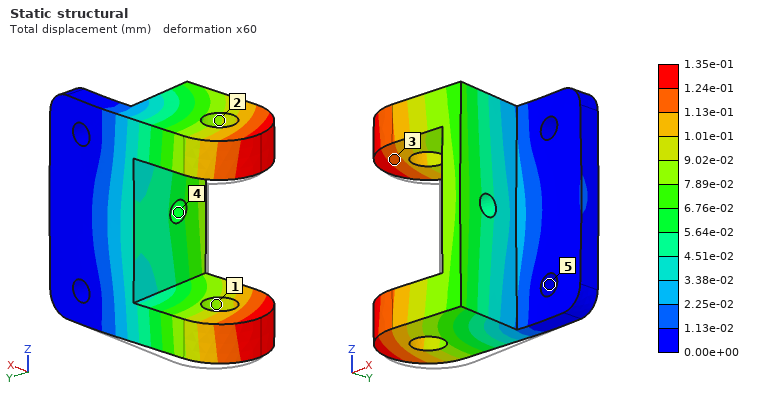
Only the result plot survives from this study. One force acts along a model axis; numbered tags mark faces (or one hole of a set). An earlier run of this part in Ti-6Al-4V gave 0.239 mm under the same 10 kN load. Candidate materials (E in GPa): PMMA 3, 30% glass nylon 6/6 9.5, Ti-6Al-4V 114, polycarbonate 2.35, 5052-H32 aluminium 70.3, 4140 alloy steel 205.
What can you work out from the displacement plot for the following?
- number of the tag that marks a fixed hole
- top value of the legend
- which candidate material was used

5
1.35e-01 mm
4140 alloy steel
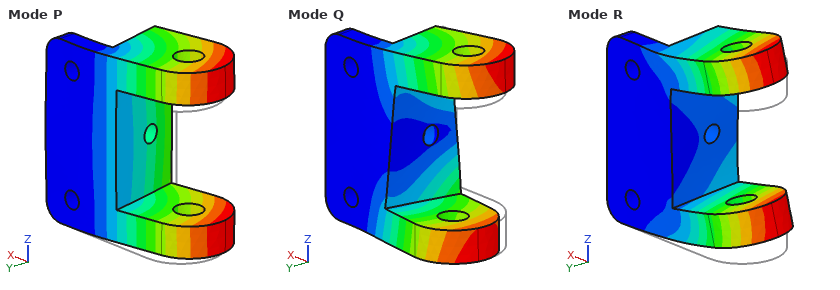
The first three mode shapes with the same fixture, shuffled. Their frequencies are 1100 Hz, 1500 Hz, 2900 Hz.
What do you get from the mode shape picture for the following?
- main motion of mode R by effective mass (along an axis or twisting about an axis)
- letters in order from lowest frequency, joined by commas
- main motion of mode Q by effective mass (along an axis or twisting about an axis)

along Z
P, Q, R
twisting about X
